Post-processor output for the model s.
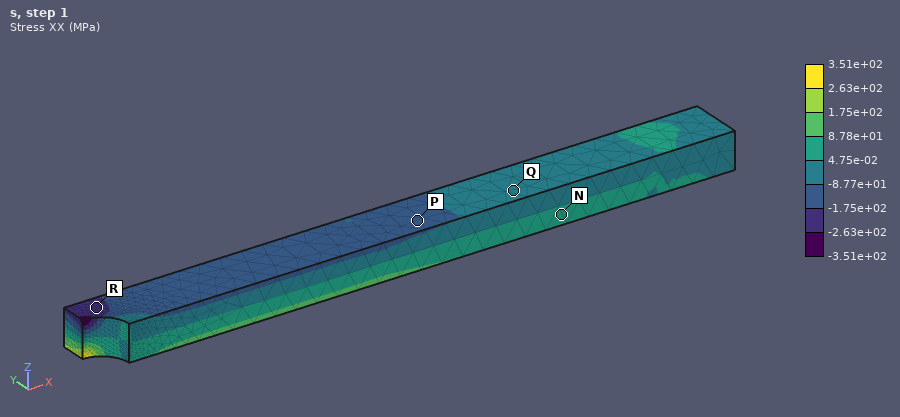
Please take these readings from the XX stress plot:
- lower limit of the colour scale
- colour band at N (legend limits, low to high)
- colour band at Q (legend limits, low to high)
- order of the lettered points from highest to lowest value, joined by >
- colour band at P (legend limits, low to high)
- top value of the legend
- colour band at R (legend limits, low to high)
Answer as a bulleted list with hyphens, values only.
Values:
- -3.51e+02 MPa
- 4.75e-02 to 8.78e+01 MPa
- -8.77e+01 to 4.75e-02 MPa
- N > Q > P > R
- -1.75e+02 to -8.77e+01 MPa
- 3.51e+02 MPa
- -2.63e+02 to -1.75e+02 MPa
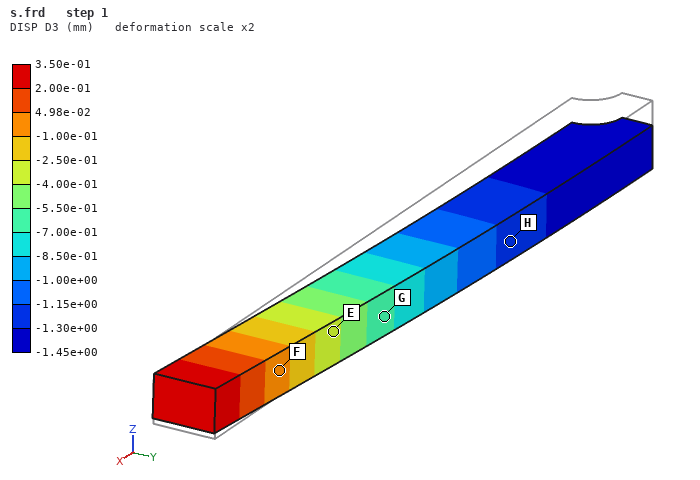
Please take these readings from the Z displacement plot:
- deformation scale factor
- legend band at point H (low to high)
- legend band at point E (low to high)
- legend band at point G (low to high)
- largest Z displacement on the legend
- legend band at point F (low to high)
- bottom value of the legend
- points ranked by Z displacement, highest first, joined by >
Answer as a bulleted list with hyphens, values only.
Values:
- 2
- -1.30e+00 to -1.15e+00 mm
- -4.00e-01 to -2.50e-01 mm
- -7.00e-01 to -5.50e-01 mm
- 3.50e-01 mm
- -1.00e-01 to 4.98e-02 mm
- -1.45e+00 mm
- F > E > G > H
